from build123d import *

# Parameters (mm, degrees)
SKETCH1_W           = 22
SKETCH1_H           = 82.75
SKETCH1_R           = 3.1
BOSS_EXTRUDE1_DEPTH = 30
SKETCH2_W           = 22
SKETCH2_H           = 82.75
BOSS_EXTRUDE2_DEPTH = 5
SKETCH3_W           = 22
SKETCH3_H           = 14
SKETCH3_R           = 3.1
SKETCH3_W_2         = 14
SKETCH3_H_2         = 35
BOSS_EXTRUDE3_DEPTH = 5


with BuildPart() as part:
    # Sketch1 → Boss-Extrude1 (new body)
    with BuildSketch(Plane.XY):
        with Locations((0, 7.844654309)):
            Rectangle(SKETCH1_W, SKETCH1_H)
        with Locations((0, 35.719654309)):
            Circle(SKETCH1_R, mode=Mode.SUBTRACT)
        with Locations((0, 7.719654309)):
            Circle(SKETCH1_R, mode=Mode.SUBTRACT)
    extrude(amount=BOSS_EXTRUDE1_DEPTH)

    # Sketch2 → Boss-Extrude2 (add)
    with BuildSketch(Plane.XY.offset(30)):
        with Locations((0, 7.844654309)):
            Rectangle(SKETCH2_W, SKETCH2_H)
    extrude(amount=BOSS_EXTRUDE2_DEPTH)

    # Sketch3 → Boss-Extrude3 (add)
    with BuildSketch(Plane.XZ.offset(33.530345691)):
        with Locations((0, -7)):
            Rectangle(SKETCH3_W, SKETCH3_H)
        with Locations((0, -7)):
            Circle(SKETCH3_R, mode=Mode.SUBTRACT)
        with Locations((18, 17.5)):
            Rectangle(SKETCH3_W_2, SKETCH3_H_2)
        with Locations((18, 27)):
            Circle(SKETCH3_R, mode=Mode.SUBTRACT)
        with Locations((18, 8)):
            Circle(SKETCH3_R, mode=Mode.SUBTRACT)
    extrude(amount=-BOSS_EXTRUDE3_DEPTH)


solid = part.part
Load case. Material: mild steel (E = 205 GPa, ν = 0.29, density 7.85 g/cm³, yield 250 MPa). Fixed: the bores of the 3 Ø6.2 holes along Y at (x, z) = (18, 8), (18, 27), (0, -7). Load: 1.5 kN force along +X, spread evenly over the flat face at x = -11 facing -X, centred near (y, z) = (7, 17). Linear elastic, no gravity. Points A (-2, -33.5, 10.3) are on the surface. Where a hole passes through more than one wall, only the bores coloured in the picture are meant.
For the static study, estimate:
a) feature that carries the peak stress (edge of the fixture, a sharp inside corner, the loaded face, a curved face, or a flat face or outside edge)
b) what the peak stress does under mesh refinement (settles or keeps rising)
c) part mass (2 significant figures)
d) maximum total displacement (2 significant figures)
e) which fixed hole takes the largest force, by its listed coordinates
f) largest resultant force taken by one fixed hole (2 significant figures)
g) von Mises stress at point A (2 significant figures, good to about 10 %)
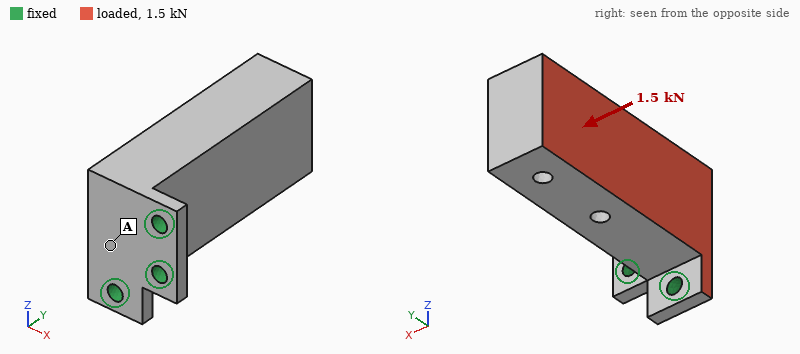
edge of the fixture
keeps rising
510 g
0.14 mm
(18, 8)
3.1 kN
25 MPa
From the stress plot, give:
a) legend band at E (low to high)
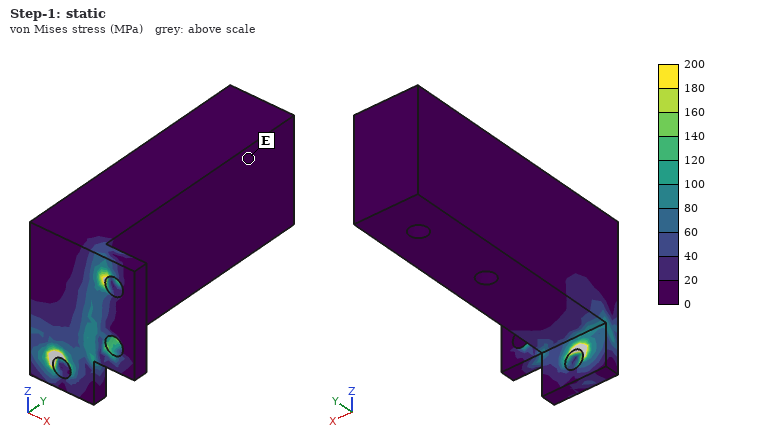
0 to 20 MPa
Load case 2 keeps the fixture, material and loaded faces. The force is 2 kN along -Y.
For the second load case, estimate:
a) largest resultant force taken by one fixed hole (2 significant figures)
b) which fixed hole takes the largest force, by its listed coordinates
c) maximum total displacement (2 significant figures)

2.0 kN
(0, -7)
0.11 mm
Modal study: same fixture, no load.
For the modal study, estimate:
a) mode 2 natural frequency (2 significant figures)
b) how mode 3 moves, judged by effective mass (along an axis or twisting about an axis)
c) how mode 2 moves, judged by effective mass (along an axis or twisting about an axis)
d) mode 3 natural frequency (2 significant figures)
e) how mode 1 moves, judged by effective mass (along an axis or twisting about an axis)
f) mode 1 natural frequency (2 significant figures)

2000 Hz
along Y
along Z
6700 Hz
along X
860 Hz
